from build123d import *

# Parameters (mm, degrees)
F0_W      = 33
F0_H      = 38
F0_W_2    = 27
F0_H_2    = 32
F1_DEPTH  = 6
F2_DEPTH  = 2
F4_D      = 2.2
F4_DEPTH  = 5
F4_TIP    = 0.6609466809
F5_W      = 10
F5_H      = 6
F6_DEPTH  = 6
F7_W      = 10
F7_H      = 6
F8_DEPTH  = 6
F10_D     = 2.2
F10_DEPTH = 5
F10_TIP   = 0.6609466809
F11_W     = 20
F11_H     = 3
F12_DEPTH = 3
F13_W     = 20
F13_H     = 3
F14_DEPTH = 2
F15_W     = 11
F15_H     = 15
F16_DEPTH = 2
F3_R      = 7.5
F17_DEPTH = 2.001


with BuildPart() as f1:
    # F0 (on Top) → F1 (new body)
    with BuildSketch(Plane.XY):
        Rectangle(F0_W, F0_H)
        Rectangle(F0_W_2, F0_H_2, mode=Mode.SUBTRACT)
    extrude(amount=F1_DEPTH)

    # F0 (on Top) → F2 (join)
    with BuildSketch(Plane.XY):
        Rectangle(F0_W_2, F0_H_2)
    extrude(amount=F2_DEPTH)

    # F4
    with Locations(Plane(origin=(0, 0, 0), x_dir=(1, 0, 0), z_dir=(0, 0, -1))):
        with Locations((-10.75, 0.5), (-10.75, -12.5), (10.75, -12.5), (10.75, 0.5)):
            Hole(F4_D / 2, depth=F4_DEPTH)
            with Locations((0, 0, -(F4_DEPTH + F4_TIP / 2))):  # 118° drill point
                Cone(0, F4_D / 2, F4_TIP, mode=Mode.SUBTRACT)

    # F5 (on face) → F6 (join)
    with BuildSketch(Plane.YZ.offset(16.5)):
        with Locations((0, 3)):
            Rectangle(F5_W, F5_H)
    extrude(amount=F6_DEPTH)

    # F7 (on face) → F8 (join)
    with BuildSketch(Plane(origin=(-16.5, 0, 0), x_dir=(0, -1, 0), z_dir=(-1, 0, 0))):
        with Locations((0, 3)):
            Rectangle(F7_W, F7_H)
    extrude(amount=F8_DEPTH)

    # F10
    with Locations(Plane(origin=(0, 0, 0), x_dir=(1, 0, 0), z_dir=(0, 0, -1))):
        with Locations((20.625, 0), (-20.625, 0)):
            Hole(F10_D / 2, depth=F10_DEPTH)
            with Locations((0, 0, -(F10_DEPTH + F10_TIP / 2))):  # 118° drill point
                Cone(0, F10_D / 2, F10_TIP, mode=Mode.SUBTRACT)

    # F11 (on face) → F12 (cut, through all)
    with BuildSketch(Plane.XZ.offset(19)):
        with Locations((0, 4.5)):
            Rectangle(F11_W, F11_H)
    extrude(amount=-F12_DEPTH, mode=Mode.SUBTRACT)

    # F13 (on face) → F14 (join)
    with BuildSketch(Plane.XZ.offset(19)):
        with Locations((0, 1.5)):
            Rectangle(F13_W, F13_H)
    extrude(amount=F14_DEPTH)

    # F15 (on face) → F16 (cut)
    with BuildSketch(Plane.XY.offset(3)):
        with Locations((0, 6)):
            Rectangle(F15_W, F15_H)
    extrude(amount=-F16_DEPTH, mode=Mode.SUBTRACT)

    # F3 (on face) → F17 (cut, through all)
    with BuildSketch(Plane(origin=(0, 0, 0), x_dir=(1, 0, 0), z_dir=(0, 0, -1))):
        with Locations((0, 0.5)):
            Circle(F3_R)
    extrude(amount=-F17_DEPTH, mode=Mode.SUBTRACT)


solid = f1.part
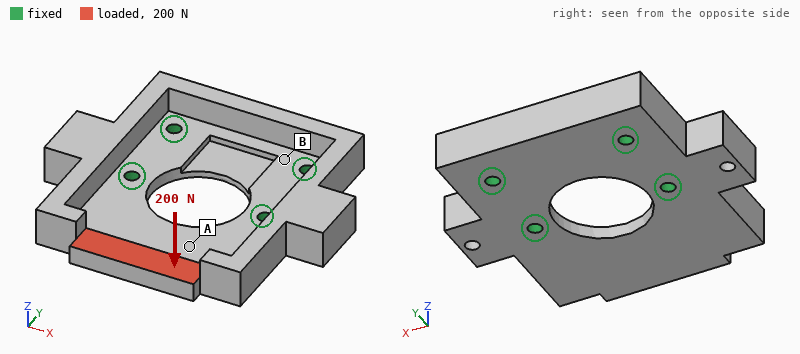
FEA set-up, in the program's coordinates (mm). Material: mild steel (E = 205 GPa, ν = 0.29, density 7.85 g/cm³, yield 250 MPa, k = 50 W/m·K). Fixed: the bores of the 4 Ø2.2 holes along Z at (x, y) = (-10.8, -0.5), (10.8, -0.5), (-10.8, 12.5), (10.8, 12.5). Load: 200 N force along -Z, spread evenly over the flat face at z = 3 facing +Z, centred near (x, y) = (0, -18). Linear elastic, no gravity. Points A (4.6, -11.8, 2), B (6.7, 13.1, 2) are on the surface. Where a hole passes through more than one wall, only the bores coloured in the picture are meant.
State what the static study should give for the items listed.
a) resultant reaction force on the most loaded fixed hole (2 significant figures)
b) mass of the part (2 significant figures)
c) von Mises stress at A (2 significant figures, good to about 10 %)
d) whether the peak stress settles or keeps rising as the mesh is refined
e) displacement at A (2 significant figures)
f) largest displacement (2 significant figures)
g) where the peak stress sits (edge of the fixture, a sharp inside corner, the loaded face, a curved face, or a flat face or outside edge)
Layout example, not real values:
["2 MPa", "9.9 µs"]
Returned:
["260 N", "33 g", "15 MPa", "keeps rising", "16 µm", "34 µm", "edge of the fixture"]
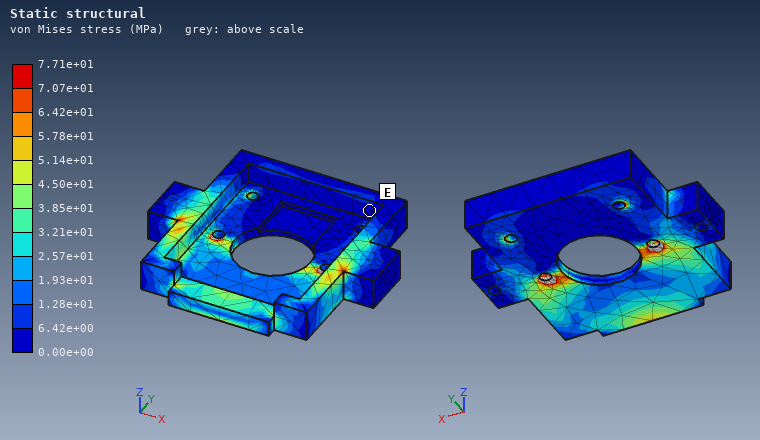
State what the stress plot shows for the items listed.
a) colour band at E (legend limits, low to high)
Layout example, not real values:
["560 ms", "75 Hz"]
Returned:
["0.00e+00 to 6.42e+00 MPa"]
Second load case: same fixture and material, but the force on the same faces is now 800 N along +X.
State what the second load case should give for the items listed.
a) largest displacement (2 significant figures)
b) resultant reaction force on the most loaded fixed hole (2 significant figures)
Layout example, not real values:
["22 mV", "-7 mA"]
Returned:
["17 µm", "640 N"]
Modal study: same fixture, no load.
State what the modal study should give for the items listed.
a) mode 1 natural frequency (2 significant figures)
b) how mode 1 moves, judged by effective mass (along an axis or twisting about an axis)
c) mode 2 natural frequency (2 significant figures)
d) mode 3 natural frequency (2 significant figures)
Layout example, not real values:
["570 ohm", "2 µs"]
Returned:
["6100 Hz", "along Z", "8200 Hz", "10000 Hz"]
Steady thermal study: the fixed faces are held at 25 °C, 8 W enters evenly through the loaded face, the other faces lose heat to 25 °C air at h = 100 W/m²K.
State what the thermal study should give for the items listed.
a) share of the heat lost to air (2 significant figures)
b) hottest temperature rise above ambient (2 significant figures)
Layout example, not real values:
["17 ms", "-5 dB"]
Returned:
["43 %", "41 K"]
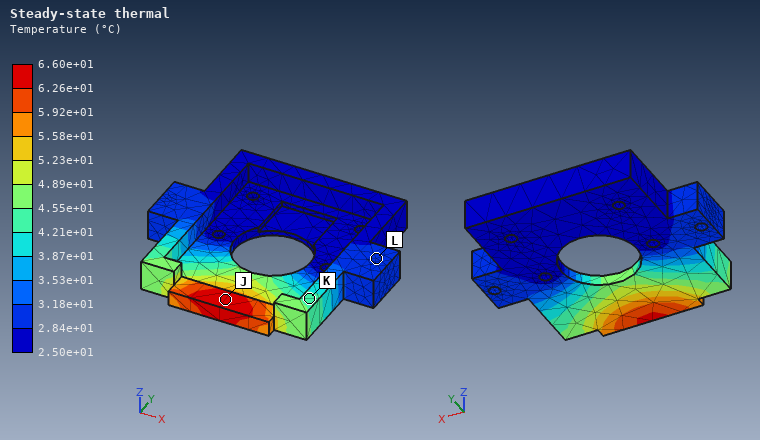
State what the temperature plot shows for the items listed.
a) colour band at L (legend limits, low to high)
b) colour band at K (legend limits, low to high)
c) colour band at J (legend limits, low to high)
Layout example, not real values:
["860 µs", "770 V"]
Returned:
["2.84e+01 to 3.18e+01 °C", "4.21e+01 to 4.55e+01 °C", "6.26e+01 to 6.60e+01 °C"]
